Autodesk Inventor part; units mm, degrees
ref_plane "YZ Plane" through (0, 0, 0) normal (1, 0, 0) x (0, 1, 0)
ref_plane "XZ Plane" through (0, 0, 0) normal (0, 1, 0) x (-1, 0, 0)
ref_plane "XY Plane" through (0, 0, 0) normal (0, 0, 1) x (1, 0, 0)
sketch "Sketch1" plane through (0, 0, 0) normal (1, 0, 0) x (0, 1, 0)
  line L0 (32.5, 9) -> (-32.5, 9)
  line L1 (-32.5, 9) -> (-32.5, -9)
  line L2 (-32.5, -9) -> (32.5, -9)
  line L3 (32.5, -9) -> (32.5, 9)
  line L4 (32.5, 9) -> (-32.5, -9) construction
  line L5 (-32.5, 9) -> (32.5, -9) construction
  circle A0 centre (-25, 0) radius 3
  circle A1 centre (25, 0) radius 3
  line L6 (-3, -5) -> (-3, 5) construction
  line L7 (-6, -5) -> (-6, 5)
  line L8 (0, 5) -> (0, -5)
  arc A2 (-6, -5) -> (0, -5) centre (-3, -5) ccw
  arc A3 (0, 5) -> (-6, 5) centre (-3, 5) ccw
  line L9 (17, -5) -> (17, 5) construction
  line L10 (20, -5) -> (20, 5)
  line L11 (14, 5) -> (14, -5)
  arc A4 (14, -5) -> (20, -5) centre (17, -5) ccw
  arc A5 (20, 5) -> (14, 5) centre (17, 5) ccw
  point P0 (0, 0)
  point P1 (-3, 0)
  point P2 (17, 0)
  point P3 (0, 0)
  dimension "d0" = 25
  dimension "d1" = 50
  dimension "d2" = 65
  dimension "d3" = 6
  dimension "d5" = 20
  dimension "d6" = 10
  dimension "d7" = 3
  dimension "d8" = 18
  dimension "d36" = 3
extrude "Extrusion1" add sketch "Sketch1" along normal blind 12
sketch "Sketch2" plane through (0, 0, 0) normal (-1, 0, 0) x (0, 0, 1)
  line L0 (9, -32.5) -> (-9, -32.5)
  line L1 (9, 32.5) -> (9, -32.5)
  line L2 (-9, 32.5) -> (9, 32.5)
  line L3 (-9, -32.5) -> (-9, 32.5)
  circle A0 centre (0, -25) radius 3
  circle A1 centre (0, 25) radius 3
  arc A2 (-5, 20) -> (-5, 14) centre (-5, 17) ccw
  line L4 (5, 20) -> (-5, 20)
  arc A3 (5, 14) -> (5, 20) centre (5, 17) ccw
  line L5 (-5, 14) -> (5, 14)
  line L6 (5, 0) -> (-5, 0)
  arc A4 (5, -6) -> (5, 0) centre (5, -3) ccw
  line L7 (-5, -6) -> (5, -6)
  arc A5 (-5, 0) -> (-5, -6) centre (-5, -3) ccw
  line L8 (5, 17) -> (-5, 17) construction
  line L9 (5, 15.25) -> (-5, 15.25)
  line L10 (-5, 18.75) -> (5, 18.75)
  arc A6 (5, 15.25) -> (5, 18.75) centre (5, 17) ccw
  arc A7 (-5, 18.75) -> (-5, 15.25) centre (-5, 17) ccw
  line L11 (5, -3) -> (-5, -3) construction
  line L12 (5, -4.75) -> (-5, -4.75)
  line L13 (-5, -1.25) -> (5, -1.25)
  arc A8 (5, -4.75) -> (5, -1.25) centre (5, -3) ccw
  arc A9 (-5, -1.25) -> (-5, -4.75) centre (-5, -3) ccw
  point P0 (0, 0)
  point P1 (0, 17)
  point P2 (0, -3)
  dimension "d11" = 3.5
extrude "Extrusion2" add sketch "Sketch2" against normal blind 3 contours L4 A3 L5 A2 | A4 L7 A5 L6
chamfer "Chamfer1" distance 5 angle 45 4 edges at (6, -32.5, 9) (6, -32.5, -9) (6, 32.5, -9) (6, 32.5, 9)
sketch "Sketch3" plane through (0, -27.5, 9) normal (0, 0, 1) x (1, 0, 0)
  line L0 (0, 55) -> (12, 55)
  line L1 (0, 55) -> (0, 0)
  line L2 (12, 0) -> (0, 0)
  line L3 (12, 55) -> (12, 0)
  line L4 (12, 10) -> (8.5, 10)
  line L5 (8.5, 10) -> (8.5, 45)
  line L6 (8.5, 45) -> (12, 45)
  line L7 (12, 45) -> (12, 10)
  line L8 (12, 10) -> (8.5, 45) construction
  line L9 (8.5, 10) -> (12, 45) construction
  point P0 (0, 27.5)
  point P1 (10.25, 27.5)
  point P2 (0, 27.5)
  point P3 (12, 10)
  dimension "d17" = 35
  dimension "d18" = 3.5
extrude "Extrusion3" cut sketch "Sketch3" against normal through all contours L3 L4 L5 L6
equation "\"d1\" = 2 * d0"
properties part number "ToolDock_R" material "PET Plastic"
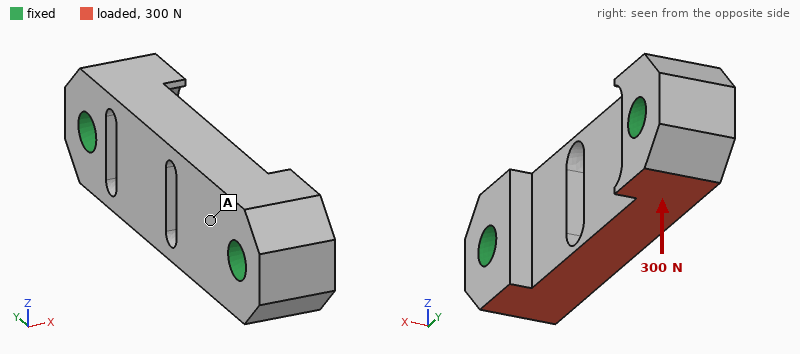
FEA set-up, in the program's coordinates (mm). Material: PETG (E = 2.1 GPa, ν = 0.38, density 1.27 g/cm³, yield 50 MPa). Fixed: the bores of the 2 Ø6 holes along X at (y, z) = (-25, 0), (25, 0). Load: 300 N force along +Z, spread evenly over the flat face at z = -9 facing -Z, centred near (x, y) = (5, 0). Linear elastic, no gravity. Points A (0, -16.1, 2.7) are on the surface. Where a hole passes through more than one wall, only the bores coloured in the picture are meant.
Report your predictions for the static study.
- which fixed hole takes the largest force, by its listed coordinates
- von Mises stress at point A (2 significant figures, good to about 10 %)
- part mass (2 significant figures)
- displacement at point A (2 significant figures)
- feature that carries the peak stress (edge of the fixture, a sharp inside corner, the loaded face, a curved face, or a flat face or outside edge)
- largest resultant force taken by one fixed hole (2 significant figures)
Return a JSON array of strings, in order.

["(-25, 0)", "1.2 MPa", "12 g", "17 µm", "a curved face", "170 N"]
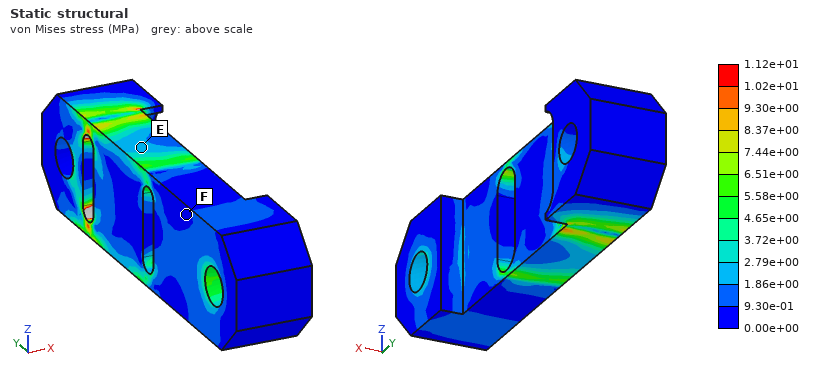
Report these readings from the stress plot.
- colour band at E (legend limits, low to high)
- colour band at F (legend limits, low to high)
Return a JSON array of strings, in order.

["1.86e+00 to 2.79e+00 MPa", "0.00e+00 to 9.30e-01 MPa"]
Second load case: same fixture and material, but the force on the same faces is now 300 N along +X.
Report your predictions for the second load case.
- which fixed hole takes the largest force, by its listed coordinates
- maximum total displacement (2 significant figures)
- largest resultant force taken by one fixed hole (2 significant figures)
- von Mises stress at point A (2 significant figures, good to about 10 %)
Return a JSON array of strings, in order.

["(-25, 0)", "0.16 mm", "170 N", "3.2 MPa"]
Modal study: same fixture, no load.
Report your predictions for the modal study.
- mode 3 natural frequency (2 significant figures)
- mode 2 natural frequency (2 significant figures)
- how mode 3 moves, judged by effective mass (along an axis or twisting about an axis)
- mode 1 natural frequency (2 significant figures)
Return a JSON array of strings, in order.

["5800 Hz", "3500 Hz", "twisting about Y", "3400 Hz"]
